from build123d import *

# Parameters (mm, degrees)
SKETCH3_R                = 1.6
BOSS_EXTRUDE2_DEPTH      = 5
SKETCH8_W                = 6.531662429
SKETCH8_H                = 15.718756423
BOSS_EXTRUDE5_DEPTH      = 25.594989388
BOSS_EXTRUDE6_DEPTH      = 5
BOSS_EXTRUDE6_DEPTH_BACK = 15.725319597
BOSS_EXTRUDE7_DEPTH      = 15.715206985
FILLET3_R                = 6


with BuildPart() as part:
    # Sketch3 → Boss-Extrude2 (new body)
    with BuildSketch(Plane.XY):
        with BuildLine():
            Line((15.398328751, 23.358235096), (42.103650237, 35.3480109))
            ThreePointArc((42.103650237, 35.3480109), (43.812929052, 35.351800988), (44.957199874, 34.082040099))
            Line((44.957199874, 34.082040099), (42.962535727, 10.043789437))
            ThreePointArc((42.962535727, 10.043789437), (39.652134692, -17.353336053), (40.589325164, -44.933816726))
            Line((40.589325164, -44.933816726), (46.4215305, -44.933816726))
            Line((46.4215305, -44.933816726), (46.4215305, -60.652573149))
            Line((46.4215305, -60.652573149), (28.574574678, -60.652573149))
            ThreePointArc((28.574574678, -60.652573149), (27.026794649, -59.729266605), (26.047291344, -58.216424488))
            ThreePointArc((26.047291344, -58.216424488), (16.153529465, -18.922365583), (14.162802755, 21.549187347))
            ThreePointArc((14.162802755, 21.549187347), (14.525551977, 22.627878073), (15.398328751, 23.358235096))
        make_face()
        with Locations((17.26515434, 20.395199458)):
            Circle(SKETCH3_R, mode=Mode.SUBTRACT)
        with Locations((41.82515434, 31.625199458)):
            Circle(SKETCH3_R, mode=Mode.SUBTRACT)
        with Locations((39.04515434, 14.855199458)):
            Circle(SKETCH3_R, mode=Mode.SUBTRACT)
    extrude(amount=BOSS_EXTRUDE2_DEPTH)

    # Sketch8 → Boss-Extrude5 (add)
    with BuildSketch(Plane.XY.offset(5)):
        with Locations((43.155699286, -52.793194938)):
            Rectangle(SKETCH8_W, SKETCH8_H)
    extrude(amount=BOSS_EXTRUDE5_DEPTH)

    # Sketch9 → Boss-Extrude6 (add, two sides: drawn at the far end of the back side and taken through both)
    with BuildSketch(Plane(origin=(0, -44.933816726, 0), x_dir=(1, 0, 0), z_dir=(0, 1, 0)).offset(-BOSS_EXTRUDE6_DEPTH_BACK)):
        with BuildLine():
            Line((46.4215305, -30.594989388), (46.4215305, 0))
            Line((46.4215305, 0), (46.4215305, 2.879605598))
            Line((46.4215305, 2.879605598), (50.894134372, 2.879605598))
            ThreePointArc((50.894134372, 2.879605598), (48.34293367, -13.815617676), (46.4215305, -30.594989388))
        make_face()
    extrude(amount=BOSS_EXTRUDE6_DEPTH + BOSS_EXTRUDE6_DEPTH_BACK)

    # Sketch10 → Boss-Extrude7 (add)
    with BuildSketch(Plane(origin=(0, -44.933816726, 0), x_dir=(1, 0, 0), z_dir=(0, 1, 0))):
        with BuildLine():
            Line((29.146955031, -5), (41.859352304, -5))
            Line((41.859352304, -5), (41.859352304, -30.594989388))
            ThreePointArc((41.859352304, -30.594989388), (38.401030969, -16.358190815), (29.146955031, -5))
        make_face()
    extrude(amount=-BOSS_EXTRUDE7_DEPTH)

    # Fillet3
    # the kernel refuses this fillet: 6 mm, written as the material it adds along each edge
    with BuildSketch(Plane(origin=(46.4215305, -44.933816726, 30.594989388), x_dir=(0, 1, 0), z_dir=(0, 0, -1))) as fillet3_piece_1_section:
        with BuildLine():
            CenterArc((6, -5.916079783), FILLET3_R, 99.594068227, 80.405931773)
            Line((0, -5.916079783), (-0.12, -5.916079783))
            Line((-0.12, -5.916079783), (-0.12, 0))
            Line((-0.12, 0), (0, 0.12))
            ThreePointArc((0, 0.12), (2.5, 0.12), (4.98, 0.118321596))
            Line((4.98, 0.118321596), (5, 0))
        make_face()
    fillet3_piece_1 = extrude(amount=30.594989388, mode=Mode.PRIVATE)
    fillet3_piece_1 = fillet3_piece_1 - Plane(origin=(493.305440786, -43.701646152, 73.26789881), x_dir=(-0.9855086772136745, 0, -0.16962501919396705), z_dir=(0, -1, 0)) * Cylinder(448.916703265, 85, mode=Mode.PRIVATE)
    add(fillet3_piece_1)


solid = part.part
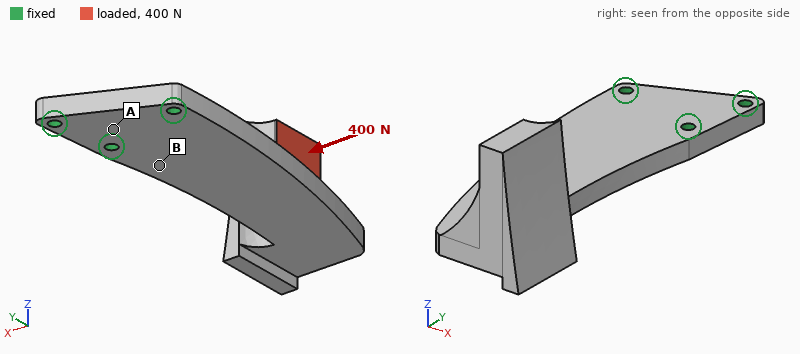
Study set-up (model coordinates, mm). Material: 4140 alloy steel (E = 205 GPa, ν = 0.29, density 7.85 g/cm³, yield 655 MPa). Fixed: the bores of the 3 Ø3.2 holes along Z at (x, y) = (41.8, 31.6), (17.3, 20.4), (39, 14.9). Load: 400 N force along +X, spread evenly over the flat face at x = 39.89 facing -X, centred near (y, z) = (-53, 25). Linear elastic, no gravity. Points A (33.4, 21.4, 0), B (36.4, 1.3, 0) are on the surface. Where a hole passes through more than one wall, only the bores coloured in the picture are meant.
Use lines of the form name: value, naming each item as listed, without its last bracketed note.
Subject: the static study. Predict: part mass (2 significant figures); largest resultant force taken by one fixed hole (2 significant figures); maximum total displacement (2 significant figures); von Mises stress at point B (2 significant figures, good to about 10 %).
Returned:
part mass: 130 g
largest resultant force taken by one fixed hole: 1.3 kN
maximum total displacement: 0.30 mm
von Mises stress at point B: 72 MPa
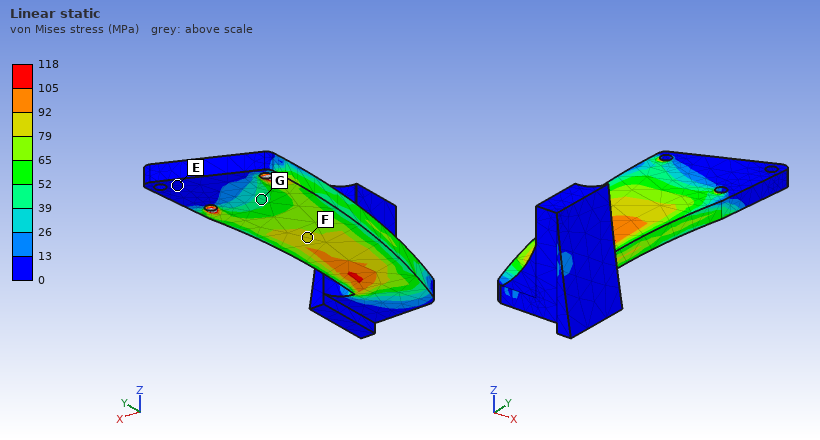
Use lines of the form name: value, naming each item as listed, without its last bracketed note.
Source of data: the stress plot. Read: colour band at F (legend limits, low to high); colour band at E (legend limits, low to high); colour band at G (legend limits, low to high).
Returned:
colour band at F: 79 to 92 MPa
colour band at E: 0 to 13 MPa
colour band at G: 39 to 52 MPa
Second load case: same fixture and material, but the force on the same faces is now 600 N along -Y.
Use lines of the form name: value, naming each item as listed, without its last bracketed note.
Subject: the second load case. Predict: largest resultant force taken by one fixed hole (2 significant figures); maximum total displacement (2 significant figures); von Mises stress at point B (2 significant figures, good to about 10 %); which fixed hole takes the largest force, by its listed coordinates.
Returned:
largest resultant force taken by one fixed hole: 650 N
maximum total displacement: 0.92 mm
von Mises stress at point B: 110 MPa
which fixed hole takes the largest force, by its listed coordinates: (39, 14.9)
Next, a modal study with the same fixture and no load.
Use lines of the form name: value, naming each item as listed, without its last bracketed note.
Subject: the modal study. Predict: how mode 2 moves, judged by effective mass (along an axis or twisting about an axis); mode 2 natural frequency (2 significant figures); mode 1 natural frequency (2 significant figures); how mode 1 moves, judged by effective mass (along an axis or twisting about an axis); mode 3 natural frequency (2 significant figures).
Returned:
how mode 2 moves, judged by effective mass: along X
mode 2 natural frequency: 1400 Hz
mode 1 natural frequency: 430 Hz
how mode 1 moves, judged by effective mass: along Z
mode 3 natural frequency: 2300 Hz
